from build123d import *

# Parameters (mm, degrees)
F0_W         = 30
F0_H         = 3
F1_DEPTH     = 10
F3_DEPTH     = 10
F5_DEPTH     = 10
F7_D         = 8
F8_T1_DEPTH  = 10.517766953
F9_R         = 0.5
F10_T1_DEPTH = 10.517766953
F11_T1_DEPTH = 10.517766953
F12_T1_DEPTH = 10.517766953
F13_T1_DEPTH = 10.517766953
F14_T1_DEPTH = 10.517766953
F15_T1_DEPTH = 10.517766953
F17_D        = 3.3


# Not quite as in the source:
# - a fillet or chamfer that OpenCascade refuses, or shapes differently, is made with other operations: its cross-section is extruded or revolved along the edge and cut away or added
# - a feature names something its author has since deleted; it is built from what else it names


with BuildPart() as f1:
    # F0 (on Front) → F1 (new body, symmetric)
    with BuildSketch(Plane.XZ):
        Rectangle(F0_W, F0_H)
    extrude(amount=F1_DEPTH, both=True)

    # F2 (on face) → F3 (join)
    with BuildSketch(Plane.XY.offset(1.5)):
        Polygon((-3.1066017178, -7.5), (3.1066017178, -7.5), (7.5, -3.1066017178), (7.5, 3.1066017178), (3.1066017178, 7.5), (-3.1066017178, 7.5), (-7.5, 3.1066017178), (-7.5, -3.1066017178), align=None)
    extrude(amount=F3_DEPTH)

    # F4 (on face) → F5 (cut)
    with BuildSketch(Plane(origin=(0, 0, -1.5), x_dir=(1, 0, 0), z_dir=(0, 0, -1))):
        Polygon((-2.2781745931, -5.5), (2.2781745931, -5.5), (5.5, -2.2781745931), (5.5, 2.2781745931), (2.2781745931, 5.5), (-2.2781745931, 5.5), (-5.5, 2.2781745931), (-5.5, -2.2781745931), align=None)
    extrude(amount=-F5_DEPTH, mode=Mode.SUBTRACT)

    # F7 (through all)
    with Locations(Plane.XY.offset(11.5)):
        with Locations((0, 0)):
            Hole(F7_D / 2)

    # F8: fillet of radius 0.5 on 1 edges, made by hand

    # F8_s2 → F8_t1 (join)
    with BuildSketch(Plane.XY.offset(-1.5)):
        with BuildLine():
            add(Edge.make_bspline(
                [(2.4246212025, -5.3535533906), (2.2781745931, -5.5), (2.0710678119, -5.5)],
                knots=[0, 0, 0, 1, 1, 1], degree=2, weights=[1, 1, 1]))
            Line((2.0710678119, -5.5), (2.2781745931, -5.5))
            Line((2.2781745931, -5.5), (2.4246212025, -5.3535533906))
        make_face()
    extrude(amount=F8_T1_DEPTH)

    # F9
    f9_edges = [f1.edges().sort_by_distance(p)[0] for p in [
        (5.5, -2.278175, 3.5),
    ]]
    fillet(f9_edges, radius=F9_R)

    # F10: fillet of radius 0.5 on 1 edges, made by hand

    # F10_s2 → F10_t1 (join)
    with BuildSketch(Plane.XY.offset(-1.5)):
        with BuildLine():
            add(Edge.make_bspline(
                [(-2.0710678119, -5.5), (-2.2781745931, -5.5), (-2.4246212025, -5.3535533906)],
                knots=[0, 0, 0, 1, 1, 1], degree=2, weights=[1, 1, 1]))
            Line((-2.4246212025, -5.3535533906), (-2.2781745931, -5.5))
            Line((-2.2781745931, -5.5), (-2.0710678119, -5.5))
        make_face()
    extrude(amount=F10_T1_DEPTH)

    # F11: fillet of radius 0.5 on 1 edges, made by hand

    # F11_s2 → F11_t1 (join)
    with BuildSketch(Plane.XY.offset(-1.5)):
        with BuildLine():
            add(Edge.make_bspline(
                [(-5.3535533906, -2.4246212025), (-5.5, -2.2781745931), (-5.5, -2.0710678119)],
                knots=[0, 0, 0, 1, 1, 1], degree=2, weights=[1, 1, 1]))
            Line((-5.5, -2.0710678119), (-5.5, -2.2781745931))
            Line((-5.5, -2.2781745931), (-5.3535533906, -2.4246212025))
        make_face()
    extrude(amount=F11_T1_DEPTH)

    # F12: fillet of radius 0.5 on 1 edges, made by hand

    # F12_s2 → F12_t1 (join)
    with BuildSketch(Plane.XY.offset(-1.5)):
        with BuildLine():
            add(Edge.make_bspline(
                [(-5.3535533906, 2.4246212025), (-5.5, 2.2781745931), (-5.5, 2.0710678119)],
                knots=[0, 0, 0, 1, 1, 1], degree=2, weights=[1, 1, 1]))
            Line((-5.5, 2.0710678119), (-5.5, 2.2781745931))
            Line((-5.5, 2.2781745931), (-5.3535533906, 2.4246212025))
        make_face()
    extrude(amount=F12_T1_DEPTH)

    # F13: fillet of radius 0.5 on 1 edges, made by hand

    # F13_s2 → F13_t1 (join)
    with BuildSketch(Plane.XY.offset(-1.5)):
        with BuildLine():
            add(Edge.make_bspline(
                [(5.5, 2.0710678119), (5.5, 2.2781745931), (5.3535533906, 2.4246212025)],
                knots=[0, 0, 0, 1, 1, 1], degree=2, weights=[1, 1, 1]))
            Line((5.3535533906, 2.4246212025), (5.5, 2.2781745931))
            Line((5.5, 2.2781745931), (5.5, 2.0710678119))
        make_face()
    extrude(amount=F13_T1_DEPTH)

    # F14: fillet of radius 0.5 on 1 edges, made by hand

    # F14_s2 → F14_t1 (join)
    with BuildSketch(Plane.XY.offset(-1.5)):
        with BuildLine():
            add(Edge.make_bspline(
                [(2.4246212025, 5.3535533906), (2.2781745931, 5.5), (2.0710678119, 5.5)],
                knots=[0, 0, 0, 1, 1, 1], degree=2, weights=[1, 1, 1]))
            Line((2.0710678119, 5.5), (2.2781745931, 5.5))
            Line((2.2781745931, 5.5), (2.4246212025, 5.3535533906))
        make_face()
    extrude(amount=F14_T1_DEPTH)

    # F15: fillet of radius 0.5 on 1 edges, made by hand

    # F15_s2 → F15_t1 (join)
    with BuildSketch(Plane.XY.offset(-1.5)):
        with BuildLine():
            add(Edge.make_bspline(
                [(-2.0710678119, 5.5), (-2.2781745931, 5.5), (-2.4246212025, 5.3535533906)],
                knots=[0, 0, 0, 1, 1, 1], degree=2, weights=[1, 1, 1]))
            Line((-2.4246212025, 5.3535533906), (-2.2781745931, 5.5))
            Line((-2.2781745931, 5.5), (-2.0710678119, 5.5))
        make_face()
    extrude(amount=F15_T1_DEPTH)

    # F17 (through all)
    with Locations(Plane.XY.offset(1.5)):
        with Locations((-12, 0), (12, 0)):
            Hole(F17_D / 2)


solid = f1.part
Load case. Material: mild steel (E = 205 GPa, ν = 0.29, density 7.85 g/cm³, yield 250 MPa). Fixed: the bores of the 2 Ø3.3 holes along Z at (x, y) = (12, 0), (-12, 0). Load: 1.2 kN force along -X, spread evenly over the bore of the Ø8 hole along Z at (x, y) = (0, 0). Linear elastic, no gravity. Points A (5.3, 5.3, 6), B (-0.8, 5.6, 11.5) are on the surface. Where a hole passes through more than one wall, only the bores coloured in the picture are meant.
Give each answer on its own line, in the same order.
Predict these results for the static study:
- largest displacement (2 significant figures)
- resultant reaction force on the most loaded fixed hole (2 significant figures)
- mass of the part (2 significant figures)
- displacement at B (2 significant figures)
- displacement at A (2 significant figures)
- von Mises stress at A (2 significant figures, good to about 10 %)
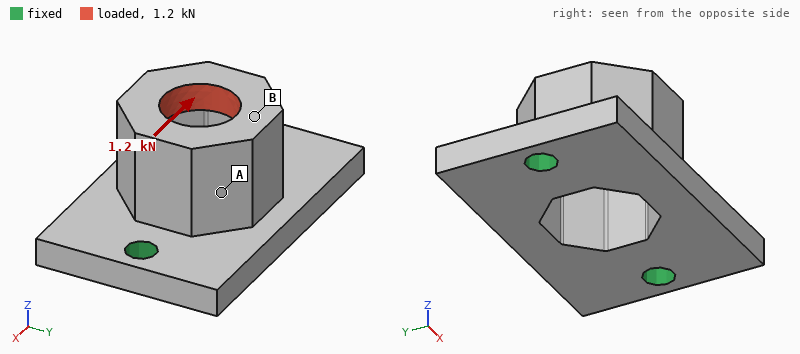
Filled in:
9.8 µm
880 N
19 g
8.1 µm
5.1 µm
28 MPa
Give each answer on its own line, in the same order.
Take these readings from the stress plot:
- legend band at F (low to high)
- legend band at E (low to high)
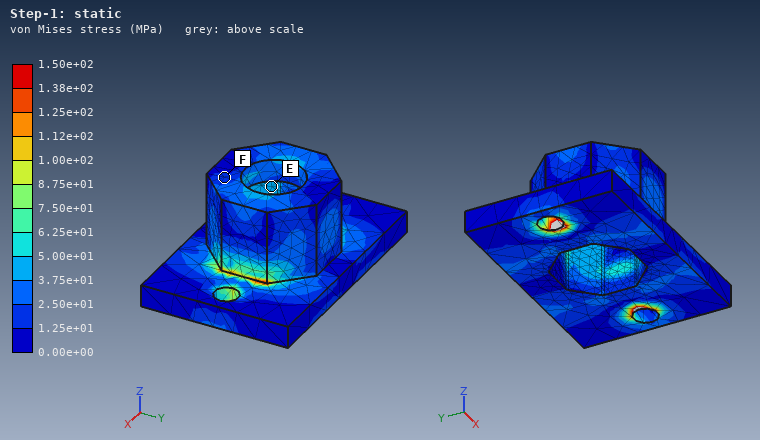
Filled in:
1.25e+01 to 2.50e+01 MPa
3.75e+01 to 5.00e+01 MPa
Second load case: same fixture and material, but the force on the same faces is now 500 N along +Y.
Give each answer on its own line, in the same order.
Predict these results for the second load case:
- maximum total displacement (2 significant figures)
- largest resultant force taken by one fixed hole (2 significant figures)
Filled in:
20 µm
250 N
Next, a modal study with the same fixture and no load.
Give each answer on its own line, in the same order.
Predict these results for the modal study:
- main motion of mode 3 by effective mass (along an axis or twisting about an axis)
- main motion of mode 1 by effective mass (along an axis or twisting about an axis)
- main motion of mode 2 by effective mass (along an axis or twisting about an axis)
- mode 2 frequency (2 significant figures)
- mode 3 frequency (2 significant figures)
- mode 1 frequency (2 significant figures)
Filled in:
along X
along Y
along Z
22 kHz
26 kHz
10 kHz
